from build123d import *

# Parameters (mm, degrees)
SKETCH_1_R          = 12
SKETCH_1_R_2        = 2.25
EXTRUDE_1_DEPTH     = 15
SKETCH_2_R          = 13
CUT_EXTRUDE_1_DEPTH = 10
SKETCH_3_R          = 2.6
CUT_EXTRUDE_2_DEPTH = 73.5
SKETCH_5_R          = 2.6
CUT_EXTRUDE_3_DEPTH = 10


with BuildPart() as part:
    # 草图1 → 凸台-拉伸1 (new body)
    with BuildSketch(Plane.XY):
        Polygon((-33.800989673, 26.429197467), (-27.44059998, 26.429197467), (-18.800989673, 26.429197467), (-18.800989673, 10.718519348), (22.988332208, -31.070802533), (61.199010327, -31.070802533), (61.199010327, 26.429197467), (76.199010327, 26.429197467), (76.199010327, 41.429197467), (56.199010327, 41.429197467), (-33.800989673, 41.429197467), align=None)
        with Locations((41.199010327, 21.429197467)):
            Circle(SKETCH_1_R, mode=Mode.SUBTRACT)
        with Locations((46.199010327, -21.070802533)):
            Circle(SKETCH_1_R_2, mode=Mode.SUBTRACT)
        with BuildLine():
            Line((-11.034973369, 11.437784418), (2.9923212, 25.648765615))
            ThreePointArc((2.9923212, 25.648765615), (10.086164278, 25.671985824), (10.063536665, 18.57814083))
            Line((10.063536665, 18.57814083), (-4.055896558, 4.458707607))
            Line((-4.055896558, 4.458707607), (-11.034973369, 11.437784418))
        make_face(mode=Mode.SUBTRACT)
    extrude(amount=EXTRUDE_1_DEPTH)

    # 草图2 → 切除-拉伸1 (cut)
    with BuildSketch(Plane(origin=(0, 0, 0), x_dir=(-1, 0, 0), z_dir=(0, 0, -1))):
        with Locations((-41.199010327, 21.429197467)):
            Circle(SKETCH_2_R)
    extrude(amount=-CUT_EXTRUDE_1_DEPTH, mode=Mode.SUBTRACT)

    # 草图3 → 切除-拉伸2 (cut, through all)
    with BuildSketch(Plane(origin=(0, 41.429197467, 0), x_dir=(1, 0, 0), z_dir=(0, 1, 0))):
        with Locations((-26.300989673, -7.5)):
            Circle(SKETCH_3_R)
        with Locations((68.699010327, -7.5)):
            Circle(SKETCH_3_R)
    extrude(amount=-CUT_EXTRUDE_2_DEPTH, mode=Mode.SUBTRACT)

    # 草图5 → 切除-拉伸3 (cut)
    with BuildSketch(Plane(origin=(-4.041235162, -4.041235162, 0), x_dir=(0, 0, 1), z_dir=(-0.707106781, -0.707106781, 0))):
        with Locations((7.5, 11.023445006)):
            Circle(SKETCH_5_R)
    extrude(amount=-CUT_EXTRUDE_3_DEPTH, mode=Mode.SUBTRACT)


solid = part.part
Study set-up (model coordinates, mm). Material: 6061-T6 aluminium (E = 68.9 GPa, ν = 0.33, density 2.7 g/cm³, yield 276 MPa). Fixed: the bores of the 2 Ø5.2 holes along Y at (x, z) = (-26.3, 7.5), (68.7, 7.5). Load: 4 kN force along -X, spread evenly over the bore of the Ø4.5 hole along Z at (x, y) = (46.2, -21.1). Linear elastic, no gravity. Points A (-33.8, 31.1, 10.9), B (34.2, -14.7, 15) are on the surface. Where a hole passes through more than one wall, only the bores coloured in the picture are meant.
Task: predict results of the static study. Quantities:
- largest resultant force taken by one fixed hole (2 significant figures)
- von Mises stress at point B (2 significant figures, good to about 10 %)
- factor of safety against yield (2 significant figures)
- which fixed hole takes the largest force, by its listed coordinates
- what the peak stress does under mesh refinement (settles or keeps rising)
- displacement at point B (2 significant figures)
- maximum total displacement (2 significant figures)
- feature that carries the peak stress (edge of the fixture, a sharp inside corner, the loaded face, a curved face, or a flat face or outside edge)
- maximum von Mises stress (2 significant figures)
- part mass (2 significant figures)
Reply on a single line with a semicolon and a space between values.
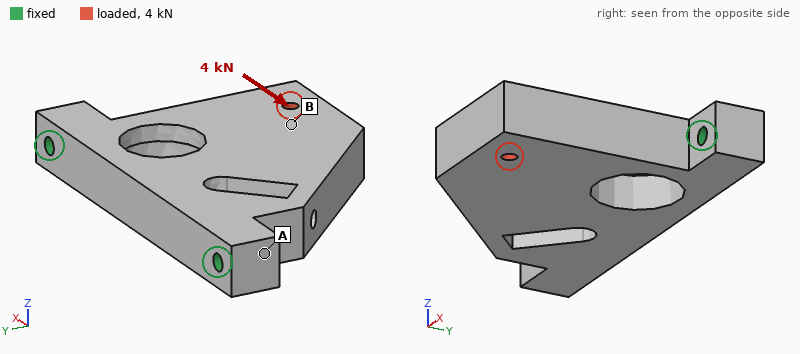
3.6 kN; 12 MPa; 2.7; (-26.3, 7.5); settles; 32 µm; 46 µm; a curved face; 100 MPa; 180 g
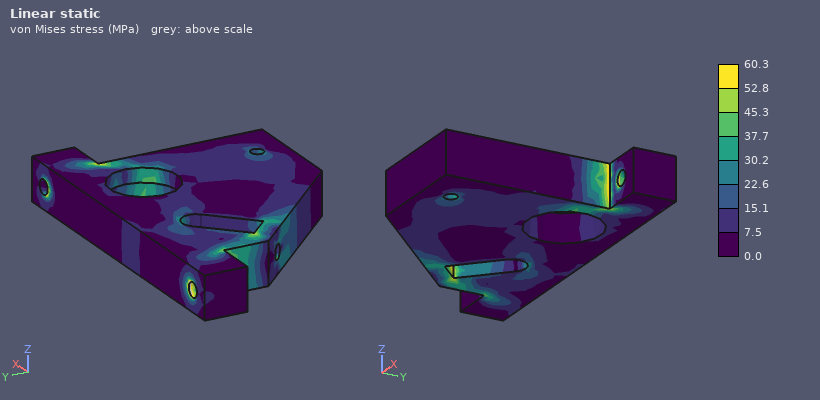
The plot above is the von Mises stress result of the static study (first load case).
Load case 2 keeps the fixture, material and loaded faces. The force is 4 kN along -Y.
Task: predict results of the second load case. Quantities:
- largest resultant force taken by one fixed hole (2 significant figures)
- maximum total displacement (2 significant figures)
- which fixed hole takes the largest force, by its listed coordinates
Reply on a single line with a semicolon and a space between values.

3.2 kN; 23 µm; (68.7, 7.5)
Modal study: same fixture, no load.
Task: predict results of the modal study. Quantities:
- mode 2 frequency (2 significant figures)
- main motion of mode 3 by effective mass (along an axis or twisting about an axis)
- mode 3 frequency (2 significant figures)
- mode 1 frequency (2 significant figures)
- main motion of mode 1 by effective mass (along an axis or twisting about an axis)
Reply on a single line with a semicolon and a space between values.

5200 Hz; along X; 6100 Hz; 1500 Hz; along Z
